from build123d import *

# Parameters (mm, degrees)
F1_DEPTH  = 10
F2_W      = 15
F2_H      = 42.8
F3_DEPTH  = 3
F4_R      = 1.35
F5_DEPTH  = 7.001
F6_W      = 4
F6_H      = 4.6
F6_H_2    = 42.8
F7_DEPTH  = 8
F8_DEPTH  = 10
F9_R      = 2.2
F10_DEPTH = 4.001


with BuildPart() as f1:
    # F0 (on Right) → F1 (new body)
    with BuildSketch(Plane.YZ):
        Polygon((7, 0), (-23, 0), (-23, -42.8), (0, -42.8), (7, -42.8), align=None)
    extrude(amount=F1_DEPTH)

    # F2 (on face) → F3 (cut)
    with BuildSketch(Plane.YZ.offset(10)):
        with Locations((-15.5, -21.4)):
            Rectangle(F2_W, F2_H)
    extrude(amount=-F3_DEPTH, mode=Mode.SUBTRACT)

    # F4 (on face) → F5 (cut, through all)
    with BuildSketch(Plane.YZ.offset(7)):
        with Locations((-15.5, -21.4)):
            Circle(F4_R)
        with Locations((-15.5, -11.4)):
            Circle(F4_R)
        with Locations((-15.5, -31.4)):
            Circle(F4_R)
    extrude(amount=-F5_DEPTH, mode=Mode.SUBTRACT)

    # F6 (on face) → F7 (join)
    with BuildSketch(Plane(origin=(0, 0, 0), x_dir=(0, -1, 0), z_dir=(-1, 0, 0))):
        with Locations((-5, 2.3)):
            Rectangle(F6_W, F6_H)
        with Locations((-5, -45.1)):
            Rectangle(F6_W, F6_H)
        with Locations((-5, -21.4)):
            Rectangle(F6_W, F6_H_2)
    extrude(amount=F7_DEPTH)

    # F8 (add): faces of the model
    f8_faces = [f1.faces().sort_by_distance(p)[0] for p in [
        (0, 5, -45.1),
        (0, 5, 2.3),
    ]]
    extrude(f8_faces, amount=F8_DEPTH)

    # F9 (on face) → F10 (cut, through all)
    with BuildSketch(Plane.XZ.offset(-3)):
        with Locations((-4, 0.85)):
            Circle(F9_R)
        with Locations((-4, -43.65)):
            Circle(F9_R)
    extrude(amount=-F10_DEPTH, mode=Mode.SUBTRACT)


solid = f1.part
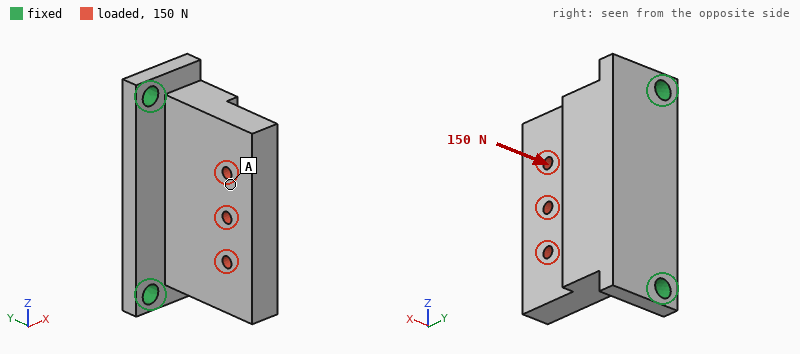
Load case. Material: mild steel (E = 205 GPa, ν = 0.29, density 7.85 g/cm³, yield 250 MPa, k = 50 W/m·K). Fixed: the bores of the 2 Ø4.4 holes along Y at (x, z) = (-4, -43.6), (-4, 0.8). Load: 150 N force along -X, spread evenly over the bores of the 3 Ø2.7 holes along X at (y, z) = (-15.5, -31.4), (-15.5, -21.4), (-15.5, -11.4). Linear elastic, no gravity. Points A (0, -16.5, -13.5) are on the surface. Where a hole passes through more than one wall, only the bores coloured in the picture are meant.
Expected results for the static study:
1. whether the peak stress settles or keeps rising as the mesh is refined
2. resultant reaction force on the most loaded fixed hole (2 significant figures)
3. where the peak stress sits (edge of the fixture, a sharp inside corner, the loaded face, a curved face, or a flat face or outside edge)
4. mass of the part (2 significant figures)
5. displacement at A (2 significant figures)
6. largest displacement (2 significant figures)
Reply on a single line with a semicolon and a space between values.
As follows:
keeps rising; 84 N; edge of the fixture; 100 g; 13 µm; 17 µm
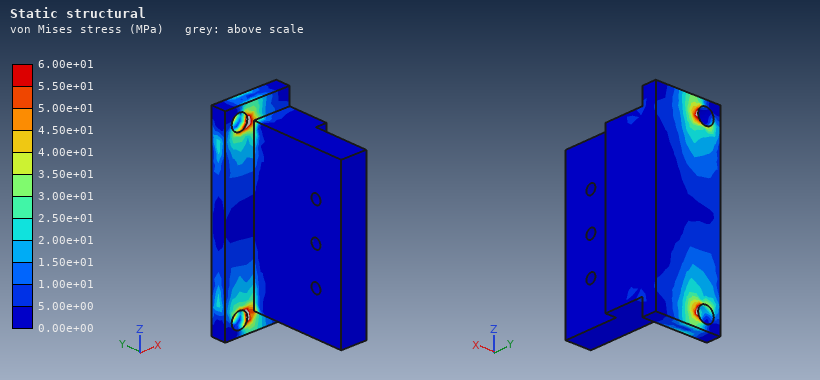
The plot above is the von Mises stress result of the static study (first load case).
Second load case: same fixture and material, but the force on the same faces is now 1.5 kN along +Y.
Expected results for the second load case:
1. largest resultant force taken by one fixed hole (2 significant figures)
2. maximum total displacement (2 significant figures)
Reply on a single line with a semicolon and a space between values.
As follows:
770 N; 34 µm
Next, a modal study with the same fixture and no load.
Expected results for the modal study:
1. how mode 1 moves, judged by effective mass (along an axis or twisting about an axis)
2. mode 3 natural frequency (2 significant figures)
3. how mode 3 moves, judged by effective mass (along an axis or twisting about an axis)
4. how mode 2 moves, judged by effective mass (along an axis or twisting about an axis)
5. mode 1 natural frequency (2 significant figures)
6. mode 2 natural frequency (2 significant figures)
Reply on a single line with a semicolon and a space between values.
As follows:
along X; 11 kHz; along Y; along Z; 2600 Hz; 9600 Hz
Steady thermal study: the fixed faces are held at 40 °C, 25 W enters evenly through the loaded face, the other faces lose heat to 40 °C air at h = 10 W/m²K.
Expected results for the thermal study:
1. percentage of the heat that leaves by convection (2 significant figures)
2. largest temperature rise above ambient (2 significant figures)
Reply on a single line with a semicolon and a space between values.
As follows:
8.0 %; 67 K
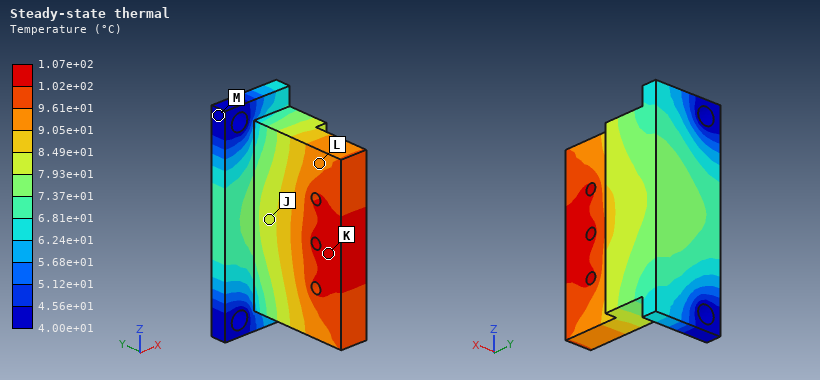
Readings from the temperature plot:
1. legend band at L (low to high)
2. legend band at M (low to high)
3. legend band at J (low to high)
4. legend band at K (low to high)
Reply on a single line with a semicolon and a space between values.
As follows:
9.05e+01 to 9.61e+01 °C; 4.00e+01 to 4.56e+01 °C; 7.93e+01 to 8.49e+01 °C; 1.02e+02 to 1.07e+02 °C
